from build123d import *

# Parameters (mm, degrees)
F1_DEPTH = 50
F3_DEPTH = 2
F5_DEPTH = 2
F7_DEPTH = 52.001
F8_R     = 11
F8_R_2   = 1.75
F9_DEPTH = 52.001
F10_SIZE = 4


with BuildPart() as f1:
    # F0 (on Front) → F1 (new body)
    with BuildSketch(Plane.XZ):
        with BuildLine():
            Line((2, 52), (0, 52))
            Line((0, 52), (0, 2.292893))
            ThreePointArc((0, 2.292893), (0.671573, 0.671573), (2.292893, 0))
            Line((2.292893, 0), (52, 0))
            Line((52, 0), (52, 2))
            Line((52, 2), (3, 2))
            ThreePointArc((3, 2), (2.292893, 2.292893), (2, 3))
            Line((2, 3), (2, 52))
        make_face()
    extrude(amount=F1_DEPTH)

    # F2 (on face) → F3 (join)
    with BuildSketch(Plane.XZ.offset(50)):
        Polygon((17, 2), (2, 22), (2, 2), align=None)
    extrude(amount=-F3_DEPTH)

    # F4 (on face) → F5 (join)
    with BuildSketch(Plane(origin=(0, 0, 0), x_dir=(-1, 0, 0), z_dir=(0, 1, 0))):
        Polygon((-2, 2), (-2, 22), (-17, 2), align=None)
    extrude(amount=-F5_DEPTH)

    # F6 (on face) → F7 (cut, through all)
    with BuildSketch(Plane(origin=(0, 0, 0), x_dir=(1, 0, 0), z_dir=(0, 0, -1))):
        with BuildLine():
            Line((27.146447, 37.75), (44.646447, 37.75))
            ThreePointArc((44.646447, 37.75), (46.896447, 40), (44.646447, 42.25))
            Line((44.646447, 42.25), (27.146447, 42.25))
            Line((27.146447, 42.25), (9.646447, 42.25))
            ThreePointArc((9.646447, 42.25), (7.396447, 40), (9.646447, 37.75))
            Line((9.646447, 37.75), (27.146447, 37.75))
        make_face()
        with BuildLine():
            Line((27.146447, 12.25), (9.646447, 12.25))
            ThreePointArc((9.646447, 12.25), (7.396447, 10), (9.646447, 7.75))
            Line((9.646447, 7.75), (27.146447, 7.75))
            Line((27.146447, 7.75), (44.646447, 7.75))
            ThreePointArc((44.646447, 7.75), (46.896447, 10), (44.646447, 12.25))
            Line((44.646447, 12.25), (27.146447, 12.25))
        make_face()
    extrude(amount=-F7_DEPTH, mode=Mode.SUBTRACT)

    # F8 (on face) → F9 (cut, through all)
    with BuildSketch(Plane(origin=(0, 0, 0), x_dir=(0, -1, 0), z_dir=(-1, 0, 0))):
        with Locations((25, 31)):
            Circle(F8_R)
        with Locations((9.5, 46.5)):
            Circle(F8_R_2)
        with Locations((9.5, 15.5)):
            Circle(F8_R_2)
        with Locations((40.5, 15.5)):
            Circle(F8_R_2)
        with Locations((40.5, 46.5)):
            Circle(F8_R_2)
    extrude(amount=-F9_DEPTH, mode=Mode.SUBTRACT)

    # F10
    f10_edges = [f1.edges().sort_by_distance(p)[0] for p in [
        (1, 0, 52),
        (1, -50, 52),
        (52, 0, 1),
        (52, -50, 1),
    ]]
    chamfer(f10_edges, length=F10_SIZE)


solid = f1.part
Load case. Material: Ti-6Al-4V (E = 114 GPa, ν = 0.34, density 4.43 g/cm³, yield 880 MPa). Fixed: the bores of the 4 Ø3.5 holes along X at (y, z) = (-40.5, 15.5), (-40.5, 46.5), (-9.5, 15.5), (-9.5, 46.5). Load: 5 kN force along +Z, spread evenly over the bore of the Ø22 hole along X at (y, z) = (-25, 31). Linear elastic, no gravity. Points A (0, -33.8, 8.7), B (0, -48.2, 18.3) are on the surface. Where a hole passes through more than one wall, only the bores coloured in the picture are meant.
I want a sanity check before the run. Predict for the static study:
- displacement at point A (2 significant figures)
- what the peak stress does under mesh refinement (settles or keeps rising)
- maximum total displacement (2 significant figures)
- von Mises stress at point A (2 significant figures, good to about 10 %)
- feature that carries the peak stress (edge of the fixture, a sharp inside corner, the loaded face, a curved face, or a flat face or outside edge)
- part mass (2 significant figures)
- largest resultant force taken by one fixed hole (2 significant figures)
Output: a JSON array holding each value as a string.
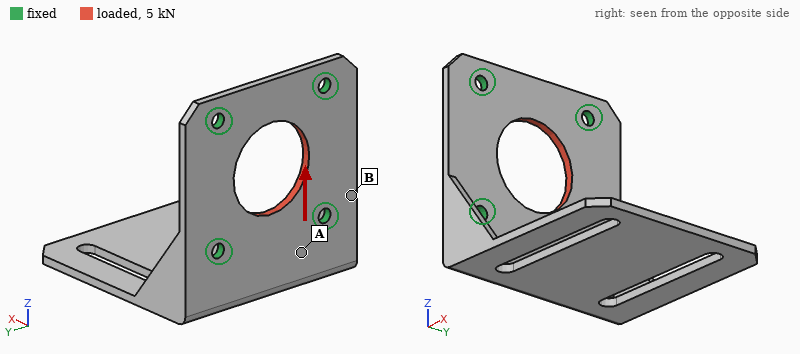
["3.7 µm", "keeps rising", "14 µm", "26 MPa", "edge of the fixture", "41 g", "1.3 kN"]
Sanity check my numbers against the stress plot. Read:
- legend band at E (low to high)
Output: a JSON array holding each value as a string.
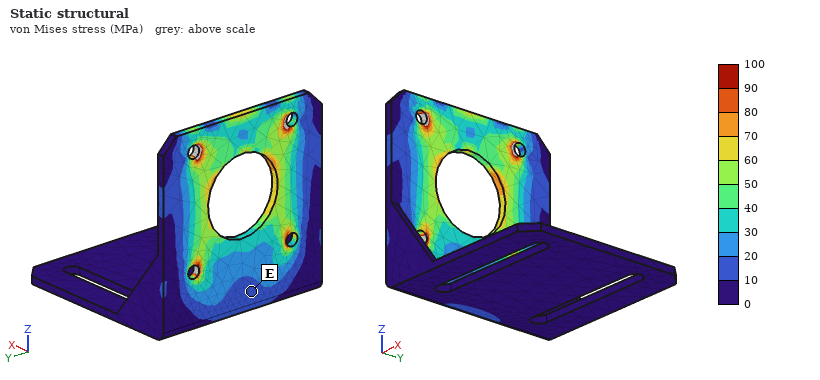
["10 to 20 MPa"]
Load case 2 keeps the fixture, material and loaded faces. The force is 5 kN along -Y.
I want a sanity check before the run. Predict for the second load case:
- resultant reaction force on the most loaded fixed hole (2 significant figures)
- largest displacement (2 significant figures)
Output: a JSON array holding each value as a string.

["1.3 kN", "10 µm"]
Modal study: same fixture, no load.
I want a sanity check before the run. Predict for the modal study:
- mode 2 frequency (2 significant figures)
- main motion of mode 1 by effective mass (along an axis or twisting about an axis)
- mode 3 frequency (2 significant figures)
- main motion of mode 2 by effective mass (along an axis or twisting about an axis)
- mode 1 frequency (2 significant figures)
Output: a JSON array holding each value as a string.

["1400 Hz", "along Z", "2300 Hz", "along Y", "670 Hz"]
